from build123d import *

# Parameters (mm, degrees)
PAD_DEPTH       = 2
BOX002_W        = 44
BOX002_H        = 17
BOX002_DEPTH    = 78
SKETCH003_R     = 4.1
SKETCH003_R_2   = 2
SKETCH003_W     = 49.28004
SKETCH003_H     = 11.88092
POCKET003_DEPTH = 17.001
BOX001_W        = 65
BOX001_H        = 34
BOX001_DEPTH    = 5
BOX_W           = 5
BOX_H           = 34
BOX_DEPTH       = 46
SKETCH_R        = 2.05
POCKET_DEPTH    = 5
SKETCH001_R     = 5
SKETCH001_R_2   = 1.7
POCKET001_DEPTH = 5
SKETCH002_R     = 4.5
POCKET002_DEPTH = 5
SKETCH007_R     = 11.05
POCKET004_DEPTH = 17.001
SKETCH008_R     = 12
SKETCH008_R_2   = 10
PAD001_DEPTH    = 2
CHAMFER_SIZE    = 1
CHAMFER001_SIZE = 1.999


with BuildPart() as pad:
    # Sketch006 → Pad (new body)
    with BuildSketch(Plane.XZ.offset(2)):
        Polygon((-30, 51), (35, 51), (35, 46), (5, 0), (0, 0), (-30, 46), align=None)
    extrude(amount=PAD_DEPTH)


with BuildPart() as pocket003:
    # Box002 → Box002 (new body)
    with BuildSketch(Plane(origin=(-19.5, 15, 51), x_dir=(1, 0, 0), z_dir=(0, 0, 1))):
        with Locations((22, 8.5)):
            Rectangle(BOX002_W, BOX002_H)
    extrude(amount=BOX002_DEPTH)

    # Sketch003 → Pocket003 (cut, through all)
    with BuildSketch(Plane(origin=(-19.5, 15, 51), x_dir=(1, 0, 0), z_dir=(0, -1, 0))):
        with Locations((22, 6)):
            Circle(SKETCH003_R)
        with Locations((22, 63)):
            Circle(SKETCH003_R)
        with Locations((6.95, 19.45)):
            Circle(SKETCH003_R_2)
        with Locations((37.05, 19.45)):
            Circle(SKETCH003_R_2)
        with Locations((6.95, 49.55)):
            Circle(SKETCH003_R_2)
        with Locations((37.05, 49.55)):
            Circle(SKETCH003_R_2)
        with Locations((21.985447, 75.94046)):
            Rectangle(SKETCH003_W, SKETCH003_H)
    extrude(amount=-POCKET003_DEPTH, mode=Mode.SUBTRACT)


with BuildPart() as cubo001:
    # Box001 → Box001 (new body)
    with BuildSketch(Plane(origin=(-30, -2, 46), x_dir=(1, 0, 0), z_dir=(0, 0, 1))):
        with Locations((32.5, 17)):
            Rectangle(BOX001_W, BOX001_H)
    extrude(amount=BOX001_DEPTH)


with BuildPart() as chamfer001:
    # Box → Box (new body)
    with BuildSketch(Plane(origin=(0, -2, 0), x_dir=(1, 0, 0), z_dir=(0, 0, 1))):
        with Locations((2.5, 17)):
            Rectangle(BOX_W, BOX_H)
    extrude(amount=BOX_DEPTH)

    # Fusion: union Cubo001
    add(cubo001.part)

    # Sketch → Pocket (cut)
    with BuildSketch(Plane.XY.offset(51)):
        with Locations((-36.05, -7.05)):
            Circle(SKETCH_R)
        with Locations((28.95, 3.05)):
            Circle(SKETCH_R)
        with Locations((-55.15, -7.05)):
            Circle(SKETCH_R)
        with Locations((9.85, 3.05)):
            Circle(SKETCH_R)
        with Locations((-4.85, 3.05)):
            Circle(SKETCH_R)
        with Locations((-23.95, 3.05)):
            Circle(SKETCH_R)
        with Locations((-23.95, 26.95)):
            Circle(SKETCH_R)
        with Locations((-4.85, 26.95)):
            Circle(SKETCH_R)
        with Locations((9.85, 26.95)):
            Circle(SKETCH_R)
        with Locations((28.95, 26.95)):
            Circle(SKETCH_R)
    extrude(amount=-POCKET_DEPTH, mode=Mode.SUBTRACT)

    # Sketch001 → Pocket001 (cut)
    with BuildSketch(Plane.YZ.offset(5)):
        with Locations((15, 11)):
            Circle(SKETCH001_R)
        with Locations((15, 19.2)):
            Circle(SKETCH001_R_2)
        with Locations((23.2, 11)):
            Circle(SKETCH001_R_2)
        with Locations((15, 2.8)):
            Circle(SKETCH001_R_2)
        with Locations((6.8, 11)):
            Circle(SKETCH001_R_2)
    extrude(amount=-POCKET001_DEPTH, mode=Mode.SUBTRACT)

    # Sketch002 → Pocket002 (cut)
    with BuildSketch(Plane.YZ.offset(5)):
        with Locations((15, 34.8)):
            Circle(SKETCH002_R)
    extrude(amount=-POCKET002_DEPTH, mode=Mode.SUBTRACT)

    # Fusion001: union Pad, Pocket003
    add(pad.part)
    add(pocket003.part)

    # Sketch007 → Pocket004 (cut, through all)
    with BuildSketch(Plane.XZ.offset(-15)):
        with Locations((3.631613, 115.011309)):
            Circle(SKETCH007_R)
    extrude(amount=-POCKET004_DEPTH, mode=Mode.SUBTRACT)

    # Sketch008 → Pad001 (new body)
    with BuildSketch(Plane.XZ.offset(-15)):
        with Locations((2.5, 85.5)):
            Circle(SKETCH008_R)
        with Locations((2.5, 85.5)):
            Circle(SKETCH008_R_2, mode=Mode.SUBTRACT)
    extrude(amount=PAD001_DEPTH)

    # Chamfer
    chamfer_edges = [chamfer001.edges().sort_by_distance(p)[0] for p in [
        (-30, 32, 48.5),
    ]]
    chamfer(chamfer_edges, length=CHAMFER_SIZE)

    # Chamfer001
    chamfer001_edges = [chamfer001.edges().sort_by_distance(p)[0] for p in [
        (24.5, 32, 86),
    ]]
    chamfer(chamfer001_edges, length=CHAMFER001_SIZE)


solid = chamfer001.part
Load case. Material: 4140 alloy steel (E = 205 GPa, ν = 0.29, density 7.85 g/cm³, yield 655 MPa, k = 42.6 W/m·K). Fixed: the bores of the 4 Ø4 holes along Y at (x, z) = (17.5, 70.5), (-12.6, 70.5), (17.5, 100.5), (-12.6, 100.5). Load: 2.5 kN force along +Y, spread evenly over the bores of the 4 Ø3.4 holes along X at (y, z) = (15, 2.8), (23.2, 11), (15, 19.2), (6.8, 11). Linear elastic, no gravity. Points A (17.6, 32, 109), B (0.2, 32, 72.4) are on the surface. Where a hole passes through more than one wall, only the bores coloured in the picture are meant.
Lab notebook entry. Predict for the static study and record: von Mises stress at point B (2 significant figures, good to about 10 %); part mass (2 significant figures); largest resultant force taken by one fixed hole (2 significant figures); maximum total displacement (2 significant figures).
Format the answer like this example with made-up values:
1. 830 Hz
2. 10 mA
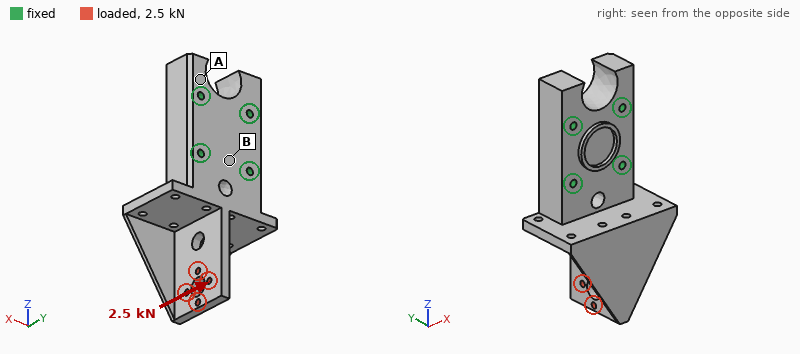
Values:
1. 30 MPa
2. 520 g
3. 1.9 kN
4. 0.15 mm
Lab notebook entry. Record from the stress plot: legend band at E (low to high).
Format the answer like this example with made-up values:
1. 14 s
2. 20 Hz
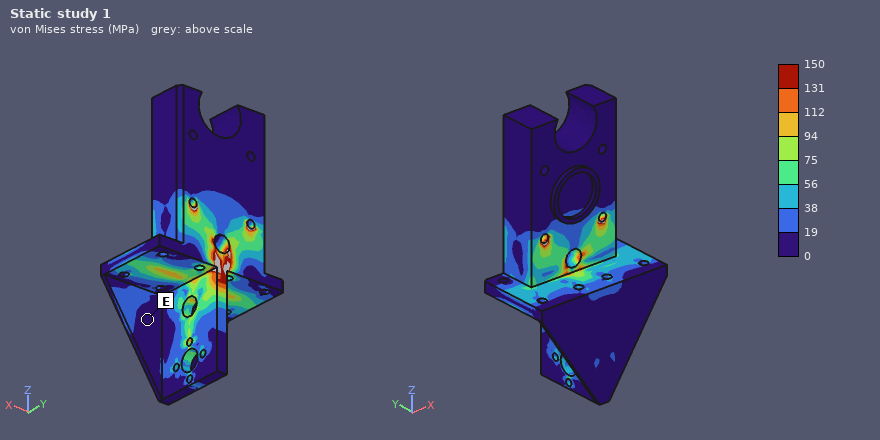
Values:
1. 0 to 19 MPa
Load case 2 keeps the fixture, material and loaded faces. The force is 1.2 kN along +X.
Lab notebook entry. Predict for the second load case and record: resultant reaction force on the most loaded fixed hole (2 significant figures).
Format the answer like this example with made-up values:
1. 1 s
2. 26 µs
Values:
1. 2.1 kN
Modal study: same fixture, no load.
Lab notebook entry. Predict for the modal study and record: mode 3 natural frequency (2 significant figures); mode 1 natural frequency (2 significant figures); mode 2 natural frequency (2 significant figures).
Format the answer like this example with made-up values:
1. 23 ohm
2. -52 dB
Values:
1. 4800 Hz
2. 2700 Hz
3. 3100 Hz
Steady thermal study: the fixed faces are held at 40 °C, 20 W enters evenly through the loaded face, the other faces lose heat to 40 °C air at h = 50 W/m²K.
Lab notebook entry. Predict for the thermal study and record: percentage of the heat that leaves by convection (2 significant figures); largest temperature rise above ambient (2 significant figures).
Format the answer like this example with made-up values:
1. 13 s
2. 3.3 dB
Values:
1. 66 %
2. 77 K
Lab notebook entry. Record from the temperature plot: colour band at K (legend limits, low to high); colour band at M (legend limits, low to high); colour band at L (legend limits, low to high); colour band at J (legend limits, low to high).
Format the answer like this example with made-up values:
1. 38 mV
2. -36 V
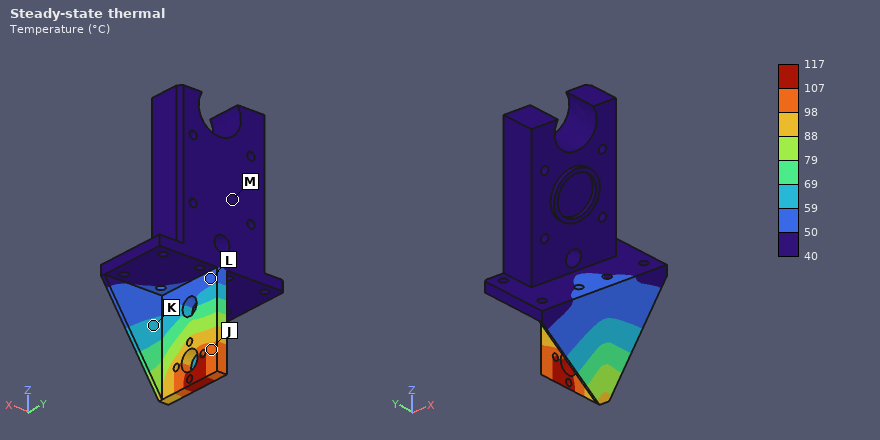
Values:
1. 59 to 69 °C
2. 40 to 50 °C
3. 50 to 59 °C
4. 98 to 107 °C
